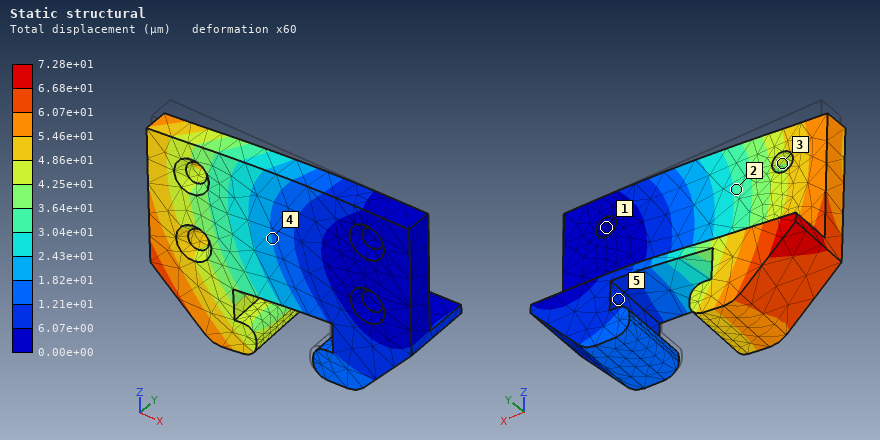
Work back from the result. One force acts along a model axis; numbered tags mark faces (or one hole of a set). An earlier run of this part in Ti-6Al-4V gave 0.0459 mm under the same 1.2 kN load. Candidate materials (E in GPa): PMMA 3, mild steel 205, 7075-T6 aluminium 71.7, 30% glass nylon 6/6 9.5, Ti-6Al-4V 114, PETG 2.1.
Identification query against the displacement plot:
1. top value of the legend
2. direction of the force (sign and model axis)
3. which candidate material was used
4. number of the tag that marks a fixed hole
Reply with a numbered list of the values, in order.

1. 7.28e+01 µm
2. -Z
3. 7075-T6 aluminium
4. 1
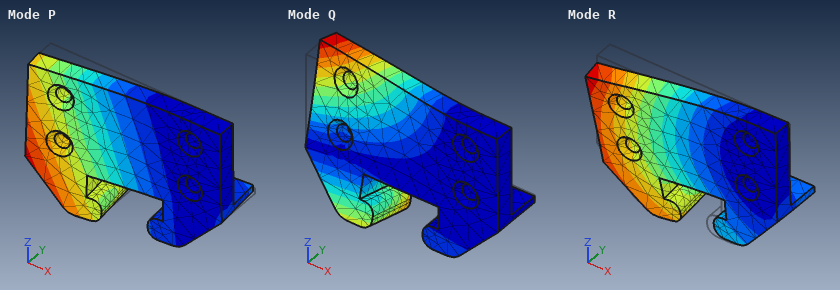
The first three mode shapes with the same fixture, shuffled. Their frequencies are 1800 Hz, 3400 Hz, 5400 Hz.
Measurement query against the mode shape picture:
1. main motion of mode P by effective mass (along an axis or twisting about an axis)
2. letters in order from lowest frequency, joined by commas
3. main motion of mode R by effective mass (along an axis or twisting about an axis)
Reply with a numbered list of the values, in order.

1. along Y
2. P, Q, R
3. along Z
